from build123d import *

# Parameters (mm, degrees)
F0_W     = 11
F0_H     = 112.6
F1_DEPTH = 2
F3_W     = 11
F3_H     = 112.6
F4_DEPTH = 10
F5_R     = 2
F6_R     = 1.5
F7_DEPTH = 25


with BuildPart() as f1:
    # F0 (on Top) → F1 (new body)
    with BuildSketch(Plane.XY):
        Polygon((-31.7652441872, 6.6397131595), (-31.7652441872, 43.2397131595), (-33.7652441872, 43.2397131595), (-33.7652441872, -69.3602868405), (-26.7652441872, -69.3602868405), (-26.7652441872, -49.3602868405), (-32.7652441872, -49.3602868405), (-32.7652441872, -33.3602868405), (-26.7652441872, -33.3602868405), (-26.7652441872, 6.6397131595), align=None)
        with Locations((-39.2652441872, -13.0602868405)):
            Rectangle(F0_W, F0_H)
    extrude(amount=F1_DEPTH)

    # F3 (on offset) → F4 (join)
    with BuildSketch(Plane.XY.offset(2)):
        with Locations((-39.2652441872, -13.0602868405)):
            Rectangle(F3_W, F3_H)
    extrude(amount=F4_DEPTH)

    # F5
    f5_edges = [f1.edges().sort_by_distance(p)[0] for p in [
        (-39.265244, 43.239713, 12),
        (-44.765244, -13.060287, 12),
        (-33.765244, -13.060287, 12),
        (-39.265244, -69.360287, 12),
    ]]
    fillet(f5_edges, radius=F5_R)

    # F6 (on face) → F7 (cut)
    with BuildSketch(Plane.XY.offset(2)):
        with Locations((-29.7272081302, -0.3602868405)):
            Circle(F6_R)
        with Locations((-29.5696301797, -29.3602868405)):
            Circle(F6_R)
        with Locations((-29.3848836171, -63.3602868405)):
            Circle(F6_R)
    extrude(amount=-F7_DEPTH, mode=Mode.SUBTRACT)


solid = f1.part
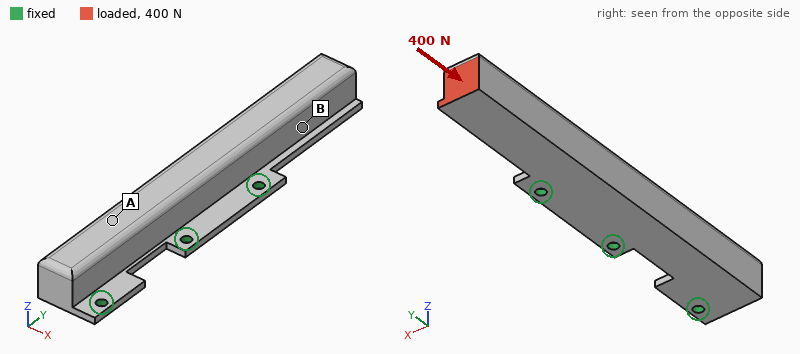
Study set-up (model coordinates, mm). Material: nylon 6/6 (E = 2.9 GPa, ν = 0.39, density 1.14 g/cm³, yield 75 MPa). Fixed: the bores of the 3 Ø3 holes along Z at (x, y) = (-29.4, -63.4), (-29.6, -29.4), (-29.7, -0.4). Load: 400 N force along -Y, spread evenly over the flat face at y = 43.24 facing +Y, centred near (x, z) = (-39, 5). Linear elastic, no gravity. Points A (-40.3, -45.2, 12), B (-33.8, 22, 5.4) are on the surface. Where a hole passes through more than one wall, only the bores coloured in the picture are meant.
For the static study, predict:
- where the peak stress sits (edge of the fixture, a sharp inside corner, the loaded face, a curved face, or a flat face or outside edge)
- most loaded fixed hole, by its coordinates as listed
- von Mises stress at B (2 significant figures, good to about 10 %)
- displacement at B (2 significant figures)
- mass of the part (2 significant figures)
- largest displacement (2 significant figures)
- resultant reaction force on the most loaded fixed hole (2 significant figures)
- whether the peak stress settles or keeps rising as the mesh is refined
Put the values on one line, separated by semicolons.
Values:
edge of the fixture; (-29.7, -0.4); 3.0 MPa; 0.088 mm; 18 g; 0.18 mm; 190 N; keeps rising
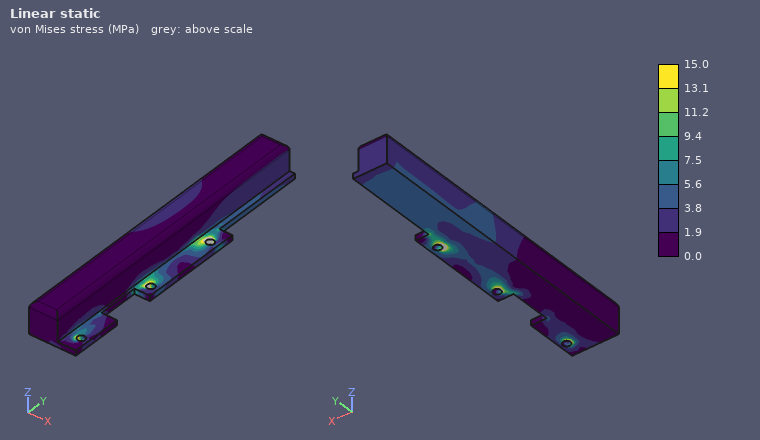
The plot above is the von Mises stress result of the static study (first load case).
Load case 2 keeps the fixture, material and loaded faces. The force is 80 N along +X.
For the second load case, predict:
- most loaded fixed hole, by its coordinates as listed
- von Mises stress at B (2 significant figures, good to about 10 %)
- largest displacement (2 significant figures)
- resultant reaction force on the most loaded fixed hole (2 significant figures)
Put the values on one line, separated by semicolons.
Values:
(-29.7, -0.4); 6.2 MPa; 1.1 mm; 210 N
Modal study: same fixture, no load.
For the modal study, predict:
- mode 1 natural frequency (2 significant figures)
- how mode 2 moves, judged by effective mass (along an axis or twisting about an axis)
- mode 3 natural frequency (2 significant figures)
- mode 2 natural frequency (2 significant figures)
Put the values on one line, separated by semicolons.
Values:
510 Hz; twisting about X; 1200 Hz; 920 Hz
